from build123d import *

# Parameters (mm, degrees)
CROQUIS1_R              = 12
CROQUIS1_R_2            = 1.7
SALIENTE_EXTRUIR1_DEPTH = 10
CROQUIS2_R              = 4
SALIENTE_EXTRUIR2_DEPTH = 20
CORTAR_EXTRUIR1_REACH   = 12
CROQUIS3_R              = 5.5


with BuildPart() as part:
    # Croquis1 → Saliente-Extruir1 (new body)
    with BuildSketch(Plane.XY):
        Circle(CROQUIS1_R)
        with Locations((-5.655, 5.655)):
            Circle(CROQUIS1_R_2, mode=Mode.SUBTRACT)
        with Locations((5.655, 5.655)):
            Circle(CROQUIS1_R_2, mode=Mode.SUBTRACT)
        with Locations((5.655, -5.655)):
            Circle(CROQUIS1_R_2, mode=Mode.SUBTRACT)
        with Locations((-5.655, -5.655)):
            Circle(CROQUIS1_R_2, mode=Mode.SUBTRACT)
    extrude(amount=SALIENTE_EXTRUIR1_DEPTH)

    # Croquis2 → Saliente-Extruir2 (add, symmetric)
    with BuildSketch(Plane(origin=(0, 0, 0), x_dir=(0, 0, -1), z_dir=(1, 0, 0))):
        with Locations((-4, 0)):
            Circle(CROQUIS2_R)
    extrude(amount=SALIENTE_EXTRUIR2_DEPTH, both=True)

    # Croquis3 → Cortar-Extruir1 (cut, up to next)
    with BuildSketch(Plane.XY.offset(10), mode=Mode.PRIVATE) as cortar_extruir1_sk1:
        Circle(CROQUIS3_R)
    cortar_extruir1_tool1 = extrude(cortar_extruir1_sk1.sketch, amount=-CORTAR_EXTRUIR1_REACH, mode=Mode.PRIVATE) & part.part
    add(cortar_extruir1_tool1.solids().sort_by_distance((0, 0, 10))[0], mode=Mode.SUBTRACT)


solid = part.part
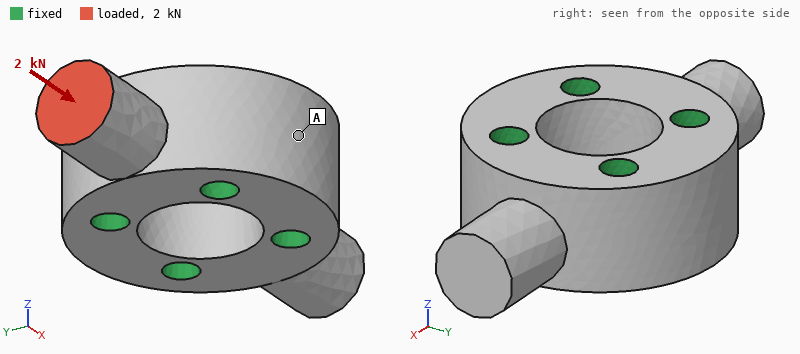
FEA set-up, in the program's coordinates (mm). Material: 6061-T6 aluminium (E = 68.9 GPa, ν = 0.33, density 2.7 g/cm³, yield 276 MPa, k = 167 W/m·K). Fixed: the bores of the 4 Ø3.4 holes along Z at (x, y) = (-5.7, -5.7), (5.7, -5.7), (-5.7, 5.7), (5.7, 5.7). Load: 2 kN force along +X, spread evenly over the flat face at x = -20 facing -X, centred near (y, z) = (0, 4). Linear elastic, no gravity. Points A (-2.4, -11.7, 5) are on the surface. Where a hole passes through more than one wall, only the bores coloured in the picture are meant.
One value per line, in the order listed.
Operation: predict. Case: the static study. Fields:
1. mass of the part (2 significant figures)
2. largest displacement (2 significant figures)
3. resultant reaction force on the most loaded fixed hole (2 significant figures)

11 g
8.8 µm
1.1 kN
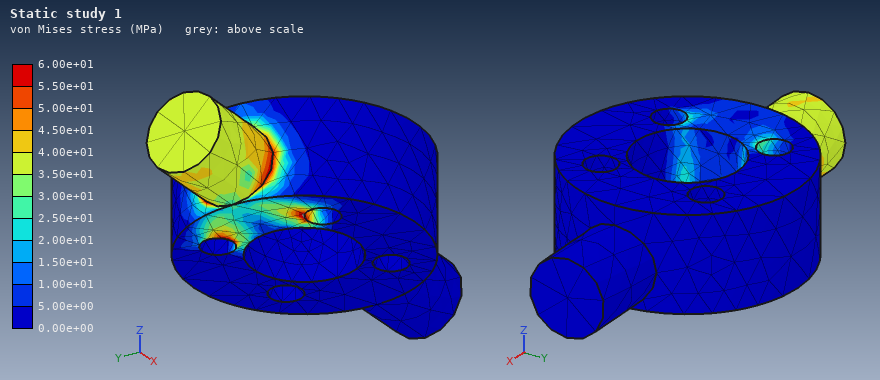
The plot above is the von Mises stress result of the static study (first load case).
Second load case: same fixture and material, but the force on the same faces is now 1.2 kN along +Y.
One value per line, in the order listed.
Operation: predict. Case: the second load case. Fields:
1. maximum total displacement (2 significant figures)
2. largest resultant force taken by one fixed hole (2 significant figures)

45 µm
1.6 kN
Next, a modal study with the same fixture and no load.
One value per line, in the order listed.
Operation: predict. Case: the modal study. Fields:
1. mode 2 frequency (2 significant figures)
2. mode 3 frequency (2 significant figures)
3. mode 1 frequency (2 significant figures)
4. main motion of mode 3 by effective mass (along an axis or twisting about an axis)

35 kHz
43 kHz
35 kHz
twisting about Z
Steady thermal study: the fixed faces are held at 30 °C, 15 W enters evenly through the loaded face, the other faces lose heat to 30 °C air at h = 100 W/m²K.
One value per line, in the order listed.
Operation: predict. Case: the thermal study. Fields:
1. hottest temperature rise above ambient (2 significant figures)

20 K
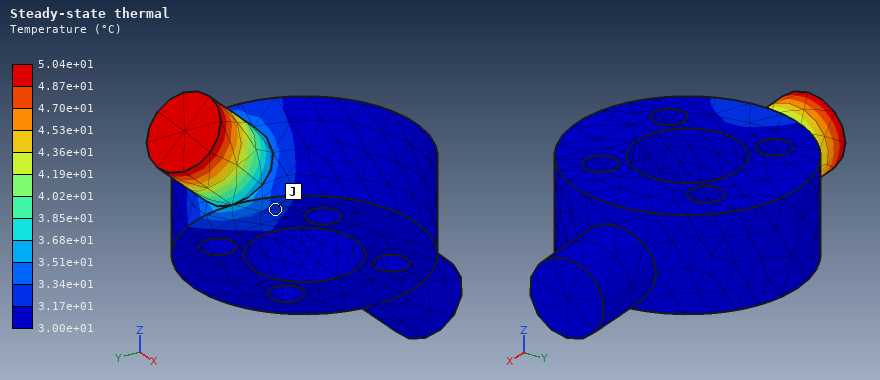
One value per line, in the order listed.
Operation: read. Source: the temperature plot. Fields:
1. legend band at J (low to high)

3.17e+01 to 3.34e+01 °C
